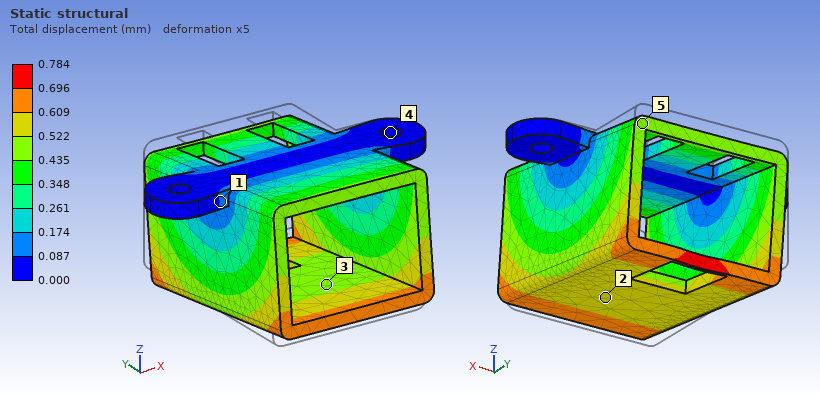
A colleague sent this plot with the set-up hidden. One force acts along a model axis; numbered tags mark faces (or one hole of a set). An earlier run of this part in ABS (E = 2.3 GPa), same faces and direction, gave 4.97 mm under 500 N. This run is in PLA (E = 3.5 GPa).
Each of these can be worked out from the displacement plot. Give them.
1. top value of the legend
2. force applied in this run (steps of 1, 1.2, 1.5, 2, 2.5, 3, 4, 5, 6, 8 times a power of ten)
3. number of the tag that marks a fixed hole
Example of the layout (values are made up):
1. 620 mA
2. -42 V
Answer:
1. 0.784 mm
2. 120 N
3. 4
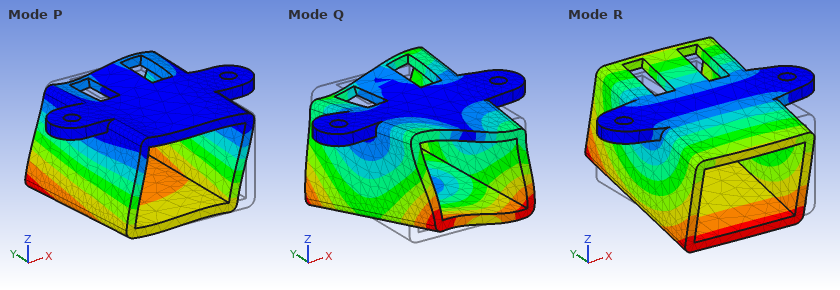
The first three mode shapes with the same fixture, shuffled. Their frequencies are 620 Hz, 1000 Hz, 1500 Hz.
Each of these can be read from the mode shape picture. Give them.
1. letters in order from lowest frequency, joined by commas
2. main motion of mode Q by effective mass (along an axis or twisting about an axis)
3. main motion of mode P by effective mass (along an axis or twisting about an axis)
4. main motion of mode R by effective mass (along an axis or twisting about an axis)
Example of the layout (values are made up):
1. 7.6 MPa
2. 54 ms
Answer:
1. R, P, Q
2. twisting about Z
3. along X
4. along Y
